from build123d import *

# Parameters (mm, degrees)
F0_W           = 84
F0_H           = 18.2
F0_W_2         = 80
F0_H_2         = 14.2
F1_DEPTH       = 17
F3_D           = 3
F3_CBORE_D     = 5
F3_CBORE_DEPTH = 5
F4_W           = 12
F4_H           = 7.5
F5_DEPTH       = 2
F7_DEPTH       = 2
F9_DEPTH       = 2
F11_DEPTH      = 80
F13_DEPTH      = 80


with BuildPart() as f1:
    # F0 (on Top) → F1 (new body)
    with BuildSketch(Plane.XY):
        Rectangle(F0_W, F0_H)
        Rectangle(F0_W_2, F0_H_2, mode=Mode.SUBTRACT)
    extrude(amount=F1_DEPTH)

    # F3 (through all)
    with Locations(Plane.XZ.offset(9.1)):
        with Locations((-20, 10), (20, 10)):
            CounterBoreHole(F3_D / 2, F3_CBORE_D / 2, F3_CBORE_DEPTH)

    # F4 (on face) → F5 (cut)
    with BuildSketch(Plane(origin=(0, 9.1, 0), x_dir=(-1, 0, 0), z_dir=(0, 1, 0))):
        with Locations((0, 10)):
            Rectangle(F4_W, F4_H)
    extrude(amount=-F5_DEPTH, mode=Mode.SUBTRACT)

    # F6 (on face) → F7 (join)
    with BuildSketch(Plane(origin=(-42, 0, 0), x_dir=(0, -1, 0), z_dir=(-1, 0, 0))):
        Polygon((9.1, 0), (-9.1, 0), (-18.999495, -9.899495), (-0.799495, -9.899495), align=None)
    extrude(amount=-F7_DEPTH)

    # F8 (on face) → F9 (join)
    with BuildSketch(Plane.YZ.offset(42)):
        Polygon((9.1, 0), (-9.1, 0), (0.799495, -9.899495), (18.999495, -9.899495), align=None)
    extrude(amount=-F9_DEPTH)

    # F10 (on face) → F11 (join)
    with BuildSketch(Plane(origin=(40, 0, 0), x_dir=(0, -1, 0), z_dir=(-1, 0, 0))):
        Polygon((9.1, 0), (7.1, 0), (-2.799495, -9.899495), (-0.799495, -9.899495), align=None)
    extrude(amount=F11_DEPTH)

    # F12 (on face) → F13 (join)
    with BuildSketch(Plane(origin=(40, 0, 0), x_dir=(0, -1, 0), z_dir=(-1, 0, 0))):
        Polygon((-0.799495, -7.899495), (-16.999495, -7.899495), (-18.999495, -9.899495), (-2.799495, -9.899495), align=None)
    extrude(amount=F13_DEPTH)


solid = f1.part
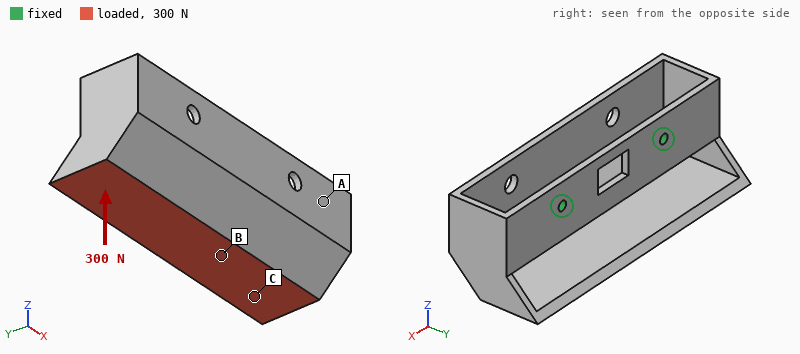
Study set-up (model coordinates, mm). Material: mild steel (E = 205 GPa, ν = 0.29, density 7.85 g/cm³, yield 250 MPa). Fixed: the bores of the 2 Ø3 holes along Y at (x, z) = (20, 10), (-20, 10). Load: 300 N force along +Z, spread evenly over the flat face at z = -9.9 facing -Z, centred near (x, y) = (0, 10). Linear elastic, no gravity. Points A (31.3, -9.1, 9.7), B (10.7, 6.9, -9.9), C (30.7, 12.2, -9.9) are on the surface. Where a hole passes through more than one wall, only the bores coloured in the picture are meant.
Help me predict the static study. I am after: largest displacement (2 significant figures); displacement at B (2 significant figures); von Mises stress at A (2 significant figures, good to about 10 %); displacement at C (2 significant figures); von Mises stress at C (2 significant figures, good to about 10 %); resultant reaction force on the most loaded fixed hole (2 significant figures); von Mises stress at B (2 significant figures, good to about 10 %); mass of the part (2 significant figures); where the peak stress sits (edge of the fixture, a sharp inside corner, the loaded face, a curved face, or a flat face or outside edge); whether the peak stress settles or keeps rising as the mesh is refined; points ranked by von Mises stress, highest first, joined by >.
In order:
0.13 mm
0.063 mm
9.7 MPa
0.050 mm
44 MPa
180 N
29 MPa
89 g
edge of the fixture
keeps rising
C > B > A
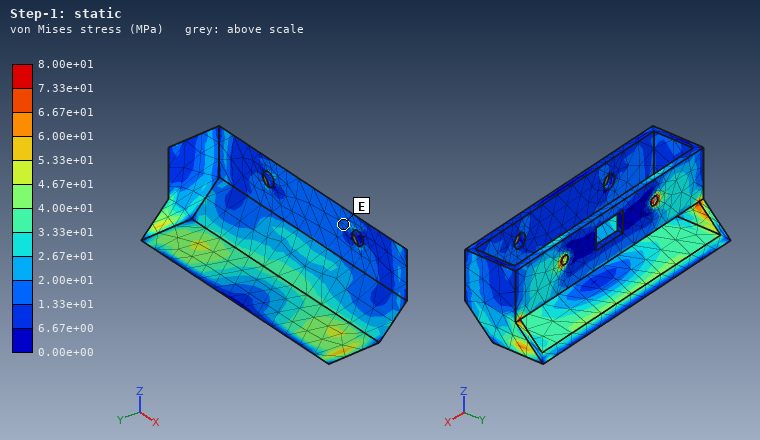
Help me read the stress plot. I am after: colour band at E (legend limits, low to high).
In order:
1.33e+01 to 2.00e+01 MPa
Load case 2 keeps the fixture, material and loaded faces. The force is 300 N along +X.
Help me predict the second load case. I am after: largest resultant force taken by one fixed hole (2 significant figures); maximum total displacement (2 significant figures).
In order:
180 N
32 µm
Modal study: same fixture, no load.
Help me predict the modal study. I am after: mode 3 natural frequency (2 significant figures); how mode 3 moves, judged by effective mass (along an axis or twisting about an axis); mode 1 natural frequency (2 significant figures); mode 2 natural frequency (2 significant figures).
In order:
1400 Hz
along Y
660 Hz
980 Hz
